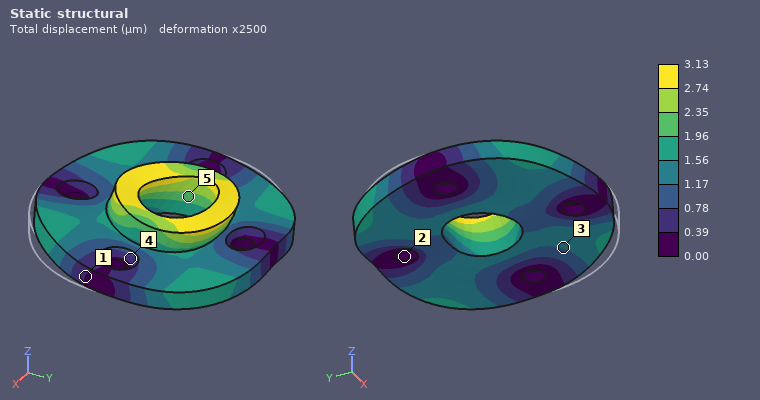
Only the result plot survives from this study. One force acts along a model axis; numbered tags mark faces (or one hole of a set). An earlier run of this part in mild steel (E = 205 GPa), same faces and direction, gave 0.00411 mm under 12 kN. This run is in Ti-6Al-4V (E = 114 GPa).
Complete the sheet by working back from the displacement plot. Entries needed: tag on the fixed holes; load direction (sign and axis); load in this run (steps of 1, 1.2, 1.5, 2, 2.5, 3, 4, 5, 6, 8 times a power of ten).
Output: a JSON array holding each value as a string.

["2", "+Y", "5 kN"]
